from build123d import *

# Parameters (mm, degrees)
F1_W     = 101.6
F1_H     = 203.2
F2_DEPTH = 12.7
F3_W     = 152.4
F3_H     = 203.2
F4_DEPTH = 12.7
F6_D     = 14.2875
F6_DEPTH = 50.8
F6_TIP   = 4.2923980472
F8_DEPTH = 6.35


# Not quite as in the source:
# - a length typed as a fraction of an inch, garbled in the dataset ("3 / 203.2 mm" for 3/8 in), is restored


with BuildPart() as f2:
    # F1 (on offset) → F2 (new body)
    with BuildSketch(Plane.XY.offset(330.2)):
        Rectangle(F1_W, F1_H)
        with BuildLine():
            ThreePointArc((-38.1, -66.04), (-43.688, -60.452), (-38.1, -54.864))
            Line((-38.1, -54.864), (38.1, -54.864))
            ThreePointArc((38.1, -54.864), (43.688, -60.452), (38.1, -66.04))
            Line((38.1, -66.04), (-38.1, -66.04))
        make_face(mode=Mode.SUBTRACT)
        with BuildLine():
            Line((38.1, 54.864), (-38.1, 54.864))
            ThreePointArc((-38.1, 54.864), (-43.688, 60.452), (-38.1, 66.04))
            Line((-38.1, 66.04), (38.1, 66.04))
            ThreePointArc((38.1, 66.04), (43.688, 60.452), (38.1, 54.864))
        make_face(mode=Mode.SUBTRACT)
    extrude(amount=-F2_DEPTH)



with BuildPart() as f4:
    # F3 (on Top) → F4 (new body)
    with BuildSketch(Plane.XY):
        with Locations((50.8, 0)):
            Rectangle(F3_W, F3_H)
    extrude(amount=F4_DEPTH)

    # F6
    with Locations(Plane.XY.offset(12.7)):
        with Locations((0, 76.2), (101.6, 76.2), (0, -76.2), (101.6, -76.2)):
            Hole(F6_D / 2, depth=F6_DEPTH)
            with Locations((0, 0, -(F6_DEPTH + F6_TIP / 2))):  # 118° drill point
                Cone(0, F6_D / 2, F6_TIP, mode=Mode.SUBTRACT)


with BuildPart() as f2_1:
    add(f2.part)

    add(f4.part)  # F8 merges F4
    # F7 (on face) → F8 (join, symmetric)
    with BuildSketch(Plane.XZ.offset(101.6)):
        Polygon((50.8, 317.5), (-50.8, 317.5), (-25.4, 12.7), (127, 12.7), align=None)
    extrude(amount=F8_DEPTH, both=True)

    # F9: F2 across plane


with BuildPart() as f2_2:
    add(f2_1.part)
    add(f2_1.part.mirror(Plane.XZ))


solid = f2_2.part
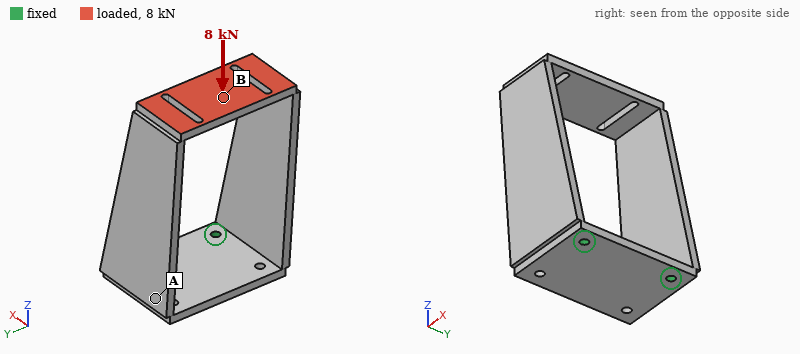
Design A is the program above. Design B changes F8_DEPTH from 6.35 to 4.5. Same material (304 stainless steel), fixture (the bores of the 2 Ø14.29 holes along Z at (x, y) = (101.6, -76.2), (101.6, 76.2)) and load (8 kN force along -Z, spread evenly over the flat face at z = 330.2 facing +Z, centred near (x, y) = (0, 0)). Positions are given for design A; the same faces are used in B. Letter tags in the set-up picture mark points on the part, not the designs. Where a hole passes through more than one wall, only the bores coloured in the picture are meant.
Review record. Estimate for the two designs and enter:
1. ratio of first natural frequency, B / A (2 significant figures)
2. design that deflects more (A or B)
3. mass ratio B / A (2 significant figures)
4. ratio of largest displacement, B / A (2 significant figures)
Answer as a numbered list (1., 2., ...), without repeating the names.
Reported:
1. 0.79
2. B
3. 0.82
4. 1.2
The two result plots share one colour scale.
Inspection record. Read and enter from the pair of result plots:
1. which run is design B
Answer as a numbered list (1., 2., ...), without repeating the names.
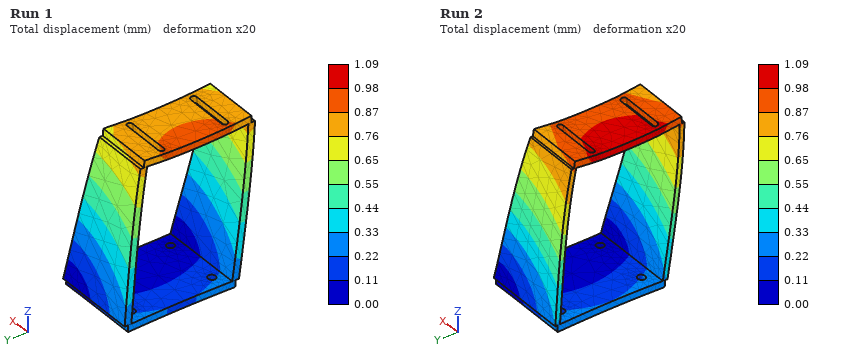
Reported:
1. Run 2
